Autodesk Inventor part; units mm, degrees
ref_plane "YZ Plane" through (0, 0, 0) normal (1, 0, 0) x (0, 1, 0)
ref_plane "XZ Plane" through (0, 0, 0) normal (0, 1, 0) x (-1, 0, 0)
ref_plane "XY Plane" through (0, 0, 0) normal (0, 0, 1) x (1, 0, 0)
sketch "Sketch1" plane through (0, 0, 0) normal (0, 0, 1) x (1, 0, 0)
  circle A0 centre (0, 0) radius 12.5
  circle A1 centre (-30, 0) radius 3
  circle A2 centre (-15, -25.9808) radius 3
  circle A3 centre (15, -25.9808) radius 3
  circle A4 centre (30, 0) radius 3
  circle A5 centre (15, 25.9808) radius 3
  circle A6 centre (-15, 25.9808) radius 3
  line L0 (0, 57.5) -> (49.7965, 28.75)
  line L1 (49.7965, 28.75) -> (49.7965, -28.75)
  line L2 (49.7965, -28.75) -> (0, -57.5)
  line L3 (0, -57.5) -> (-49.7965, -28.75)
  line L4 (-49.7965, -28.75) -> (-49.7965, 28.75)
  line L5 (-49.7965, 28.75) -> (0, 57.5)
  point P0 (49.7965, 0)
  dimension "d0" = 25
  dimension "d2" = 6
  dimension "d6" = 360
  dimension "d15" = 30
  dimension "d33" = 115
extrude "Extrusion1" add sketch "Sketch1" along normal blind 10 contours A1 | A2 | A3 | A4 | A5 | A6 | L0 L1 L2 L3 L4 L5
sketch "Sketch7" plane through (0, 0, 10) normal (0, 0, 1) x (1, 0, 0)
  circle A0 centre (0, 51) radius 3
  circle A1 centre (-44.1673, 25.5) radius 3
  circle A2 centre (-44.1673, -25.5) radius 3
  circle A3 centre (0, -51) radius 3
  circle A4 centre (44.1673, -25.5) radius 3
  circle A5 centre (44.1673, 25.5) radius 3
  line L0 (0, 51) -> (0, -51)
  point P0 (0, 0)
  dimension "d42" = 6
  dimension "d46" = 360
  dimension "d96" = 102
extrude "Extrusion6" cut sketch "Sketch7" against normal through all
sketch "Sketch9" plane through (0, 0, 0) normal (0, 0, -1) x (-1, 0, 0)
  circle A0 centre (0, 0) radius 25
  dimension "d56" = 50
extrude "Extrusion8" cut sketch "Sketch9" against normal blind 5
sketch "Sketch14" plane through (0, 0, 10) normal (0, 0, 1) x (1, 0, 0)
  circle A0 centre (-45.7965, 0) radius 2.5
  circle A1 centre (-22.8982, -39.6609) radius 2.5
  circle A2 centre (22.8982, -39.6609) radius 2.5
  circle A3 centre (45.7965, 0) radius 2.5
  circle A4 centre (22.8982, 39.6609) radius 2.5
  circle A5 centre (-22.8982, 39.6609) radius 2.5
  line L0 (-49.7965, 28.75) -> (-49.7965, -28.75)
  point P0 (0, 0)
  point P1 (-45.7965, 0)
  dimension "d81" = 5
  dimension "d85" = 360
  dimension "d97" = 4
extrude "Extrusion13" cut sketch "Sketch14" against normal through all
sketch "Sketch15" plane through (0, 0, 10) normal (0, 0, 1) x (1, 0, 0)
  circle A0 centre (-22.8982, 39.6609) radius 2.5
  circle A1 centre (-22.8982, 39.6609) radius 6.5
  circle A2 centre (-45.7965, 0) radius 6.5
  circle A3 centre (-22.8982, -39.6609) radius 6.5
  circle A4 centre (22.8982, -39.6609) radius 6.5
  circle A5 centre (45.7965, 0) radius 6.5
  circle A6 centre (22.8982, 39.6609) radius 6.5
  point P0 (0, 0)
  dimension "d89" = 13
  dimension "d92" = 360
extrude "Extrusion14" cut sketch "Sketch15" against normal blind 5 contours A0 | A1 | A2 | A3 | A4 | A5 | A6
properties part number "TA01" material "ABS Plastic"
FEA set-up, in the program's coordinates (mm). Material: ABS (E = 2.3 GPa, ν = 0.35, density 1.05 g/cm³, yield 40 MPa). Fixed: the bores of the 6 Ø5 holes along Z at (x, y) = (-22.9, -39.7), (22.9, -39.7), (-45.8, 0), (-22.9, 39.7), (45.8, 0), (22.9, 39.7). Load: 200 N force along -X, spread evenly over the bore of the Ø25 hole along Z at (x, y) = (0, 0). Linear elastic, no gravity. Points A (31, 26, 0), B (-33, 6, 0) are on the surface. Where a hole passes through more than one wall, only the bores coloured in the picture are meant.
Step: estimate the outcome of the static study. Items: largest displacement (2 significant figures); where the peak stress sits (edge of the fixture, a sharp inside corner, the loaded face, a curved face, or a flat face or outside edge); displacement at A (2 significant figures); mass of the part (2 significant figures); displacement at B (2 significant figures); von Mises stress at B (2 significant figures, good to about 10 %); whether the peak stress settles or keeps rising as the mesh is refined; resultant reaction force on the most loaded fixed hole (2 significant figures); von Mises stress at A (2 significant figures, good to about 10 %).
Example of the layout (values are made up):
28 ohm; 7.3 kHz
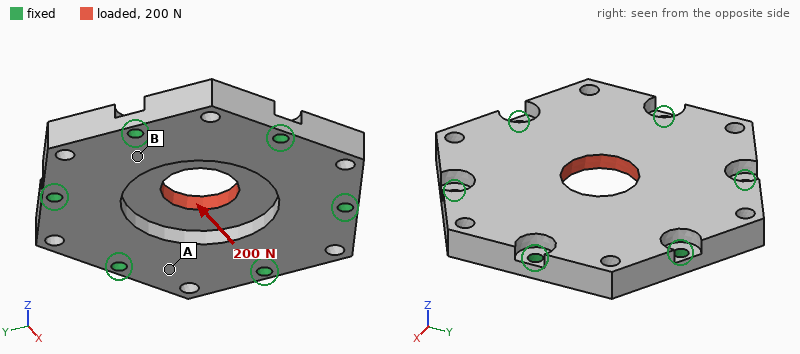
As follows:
11 µm; edge of the fixture; 1.8 µm; 71 g; 2.6 µm; 0.20 MPa; keeps rising; 44 N; 0.11 MPa
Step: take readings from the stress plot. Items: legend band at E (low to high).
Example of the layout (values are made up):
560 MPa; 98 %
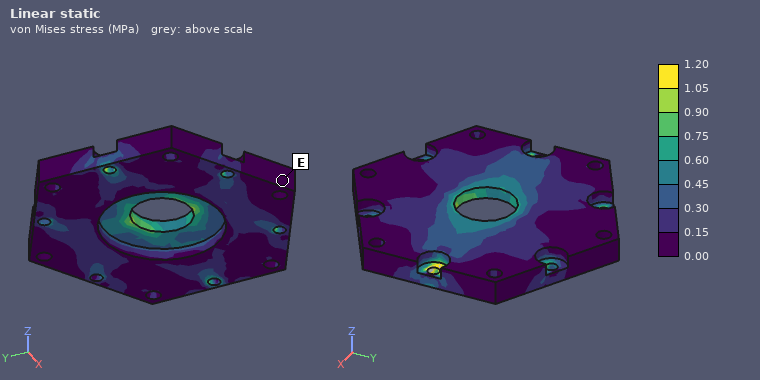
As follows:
0.00 to 0.15 MPa
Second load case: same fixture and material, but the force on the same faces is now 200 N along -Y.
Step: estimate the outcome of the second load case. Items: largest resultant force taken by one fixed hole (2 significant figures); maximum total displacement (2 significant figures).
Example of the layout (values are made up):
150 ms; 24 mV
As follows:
40 N; 11 µm
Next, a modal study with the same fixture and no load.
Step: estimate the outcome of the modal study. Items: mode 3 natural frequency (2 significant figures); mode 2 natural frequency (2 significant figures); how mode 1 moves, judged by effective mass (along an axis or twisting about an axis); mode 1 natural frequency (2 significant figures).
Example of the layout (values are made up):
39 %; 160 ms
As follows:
3400 Hz; 3400 Hz; along Z; 2300 Hz
